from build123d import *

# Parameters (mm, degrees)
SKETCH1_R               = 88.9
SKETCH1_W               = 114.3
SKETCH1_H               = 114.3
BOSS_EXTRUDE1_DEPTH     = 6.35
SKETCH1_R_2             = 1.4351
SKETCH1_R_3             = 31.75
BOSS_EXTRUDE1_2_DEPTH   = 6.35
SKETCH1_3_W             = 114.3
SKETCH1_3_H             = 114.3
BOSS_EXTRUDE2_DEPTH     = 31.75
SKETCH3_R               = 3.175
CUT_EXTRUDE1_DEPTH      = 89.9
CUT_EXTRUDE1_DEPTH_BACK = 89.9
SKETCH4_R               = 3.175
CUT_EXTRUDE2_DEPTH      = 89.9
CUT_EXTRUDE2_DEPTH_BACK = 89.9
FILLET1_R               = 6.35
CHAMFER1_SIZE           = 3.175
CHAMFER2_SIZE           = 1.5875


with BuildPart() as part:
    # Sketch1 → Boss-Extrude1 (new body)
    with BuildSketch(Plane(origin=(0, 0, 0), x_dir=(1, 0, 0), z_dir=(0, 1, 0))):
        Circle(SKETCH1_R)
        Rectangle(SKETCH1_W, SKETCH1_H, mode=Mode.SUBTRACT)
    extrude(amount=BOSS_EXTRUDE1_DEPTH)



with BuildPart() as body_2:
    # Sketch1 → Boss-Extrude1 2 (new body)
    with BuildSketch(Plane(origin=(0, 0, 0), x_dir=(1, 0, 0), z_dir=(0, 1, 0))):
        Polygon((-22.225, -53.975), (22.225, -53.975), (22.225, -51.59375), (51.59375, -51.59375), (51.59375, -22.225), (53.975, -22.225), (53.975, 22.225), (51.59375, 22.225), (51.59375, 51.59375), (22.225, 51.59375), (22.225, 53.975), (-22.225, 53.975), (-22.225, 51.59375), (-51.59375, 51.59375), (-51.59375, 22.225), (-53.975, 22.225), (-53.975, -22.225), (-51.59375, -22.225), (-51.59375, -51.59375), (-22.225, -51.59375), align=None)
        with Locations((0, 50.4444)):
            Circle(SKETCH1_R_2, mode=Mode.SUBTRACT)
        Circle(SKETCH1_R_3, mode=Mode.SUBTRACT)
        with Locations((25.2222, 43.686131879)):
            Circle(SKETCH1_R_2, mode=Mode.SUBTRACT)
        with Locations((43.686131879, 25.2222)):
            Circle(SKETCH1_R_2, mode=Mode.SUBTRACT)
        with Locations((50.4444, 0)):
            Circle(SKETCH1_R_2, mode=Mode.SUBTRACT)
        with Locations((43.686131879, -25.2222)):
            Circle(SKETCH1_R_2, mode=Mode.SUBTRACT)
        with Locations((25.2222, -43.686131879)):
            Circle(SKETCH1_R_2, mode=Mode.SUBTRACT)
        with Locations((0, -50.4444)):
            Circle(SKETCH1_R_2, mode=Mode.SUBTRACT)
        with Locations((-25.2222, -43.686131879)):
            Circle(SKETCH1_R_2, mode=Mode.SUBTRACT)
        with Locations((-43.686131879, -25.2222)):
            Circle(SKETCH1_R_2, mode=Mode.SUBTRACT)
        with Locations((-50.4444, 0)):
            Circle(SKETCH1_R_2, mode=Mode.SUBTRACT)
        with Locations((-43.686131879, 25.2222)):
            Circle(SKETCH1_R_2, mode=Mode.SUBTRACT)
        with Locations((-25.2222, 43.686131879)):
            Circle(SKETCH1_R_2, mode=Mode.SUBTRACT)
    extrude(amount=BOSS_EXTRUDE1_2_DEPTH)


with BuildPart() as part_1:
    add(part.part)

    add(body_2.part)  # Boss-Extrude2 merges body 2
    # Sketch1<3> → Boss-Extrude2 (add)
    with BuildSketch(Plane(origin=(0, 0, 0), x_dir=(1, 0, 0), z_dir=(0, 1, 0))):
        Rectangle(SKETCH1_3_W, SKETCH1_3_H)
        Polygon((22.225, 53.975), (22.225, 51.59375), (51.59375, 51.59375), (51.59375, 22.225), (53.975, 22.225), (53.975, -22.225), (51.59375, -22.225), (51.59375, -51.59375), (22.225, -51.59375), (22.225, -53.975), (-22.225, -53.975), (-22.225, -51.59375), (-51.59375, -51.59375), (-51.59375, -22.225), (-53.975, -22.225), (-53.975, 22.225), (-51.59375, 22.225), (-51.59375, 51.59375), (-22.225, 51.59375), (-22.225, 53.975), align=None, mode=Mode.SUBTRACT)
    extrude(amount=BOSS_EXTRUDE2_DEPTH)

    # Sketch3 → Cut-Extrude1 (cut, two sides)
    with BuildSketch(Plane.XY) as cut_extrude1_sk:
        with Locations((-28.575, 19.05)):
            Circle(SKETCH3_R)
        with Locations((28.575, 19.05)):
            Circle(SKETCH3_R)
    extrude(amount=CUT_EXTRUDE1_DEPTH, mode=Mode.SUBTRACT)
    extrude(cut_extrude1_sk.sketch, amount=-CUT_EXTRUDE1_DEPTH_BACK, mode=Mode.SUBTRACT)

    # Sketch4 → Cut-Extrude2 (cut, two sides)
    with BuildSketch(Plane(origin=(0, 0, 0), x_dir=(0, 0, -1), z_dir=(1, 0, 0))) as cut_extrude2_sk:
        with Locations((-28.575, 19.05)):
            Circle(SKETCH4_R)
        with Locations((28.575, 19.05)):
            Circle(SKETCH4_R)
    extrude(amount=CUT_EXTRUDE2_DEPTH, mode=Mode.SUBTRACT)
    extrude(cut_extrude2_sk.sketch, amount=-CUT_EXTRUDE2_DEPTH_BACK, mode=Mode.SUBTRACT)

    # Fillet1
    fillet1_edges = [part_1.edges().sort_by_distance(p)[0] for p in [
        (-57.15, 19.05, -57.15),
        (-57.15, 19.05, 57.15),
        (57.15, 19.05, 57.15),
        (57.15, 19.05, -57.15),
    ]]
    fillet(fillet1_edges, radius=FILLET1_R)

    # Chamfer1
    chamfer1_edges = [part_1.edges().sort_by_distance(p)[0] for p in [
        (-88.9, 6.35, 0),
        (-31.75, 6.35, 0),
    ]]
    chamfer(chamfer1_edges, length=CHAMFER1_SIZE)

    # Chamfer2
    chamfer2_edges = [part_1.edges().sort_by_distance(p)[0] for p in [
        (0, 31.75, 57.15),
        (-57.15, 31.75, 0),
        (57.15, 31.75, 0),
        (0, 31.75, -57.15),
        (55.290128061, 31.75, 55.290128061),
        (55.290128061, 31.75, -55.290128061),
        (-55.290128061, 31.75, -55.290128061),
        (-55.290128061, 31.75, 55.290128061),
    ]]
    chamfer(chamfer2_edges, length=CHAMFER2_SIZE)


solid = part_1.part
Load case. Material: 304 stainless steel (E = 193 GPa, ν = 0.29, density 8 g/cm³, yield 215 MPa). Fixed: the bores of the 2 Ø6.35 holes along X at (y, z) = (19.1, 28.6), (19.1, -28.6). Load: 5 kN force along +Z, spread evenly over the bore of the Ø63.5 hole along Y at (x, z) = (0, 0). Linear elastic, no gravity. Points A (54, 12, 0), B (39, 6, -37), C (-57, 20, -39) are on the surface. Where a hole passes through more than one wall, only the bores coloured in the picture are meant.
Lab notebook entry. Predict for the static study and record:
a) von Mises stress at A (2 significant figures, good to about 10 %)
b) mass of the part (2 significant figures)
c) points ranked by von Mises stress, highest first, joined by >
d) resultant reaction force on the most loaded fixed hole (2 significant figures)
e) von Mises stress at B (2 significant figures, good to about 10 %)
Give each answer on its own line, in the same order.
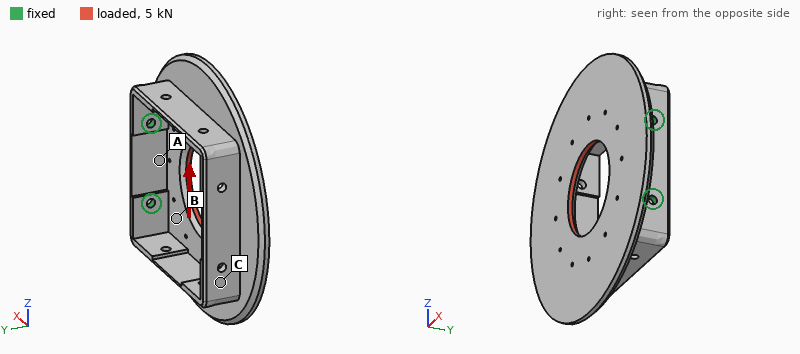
45 MPa
1.4 kg
A > B > C
5.0 kN
24 MPa
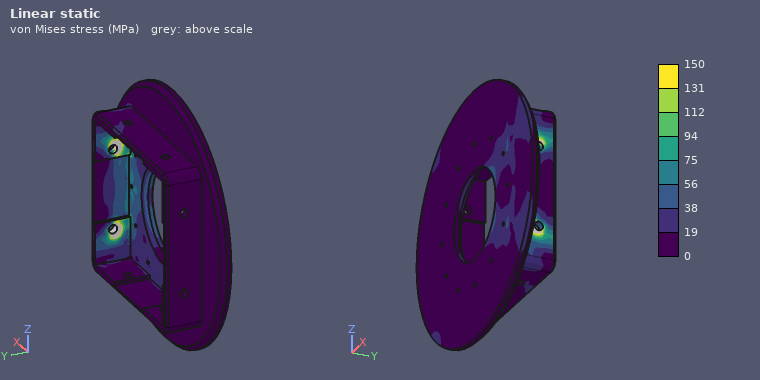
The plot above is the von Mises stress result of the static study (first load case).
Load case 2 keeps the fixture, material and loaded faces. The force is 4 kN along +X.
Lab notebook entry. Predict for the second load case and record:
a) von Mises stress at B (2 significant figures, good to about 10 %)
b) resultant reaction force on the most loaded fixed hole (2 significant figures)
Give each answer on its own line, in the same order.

14 MPa
2.0 kN
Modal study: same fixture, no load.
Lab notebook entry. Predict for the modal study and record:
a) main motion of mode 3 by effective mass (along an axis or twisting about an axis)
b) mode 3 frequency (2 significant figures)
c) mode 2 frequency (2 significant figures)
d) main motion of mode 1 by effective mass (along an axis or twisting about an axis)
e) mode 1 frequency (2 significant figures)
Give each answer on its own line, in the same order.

along Z
930 Hz
520 Hz
along Y
240 Hz
